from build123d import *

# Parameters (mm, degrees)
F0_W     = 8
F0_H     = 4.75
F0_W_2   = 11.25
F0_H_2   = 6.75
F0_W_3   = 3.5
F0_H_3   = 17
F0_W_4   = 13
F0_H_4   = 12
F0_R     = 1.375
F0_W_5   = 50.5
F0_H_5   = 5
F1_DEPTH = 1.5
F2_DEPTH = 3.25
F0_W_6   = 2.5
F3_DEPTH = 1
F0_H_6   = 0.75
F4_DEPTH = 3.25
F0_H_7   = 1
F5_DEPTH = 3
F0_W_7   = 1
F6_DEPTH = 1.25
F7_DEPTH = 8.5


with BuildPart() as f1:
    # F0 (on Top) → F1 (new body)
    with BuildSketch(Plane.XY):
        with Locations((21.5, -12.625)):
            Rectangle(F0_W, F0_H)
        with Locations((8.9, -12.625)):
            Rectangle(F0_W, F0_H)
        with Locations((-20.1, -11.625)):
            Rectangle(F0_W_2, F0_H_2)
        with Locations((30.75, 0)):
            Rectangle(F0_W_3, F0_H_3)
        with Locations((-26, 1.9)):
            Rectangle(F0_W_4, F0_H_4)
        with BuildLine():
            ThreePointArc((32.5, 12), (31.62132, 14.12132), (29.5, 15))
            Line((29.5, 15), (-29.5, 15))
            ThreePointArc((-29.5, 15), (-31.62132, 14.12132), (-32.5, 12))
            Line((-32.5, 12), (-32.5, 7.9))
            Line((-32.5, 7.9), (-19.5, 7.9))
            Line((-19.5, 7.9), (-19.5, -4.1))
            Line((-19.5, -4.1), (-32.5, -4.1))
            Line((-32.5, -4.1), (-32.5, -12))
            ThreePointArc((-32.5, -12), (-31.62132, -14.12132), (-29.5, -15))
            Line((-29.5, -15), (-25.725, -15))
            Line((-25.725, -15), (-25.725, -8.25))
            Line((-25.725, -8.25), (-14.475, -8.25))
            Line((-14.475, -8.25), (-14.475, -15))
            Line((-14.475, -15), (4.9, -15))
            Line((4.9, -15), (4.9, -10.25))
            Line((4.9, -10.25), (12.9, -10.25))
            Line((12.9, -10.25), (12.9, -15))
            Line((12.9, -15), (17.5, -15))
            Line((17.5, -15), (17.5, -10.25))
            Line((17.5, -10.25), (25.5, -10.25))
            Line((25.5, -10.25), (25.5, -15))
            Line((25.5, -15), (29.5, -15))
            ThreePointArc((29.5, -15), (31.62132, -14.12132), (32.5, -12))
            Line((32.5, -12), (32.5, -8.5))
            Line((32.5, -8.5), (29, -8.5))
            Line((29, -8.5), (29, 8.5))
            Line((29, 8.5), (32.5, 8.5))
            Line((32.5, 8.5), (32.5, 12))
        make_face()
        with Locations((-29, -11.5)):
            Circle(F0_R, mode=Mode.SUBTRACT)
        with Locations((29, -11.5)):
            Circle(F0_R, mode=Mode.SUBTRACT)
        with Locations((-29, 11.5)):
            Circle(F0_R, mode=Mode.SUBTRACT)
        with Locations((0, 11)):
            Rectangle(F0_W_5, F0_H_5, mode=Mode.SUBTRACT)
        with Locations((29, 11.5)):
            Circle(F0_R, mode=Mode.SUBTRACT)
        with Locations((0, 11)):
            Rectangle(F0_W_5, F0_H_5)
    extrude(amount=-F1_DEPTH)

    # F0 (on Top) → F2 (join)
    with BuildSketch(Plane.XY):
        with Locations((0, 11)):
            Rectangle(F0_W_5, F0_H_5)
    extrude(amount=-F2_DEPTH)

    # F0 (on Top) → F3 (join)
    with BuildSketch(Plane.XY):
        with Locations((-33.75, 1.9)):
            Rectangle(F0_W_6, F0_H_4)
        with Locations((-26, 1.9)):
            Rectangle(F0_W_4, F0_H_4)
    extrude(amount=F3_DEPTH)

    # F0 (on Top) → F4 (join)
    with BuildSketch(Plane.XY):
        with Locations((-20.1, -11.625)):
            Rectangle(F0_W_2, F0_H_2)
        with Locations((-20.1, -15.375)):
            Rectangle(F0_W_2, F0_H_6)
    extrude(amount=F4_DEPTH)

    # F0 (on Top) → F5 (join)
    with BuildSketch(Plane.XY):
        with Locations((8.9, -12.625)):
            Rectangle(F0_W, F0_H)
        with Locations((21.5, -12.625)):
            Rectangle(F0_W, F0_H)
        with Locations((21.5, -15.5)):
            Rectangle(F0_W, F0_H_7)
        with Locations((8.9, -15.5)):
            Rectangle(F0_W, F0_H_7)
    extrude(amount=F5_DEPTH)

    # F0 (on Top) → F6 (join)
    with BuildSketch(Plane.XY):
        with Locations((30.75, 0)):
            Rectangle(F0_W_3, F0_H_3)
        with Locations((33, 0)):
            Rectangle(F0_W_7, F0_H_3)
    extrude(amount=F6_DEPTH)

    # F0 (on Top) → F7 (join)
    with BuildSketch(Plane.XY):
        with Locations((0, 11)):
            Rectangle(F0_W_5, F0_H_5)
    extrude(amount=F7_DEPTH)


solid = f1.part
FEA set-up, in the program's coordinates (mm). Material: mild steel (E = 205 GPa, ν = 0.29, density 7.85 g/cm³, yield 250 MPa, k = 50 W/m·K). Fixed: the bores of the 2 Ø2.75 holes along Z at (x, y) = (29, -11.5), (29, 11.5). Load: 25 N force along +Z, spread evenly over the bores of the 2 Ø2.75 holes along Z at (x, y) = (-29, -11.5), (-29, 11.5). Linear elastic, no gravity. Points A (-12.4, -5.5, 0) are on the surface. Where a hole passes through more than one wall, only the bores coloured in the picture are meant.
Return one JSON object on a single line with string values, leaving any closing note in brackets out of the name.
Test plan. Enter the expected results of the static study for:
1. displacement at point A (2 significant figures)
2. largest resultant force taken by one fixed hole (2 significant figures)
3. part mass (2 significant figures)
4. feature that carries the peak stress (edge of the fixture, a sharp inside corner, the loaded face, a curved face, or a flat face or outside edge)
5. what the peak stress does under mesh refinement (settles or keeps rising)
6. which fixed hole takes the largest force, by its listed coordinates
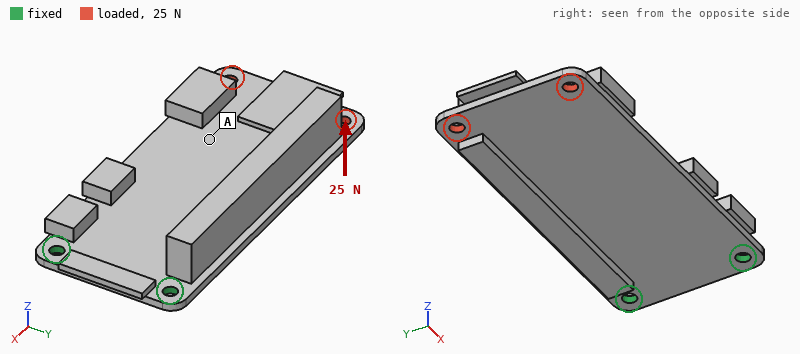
{"displacement at point A": "0.20 mm", "largest resultant force taken by one fixed hole": "21 N", "part mass": "49 g", "feature that carries the peak stress": "edge of the fixture", "what the peak stress does under mesh refinement": "keeps rising", "which fixed hole takes the largest force, by its listed coordinates": "(29, -11.5)"}
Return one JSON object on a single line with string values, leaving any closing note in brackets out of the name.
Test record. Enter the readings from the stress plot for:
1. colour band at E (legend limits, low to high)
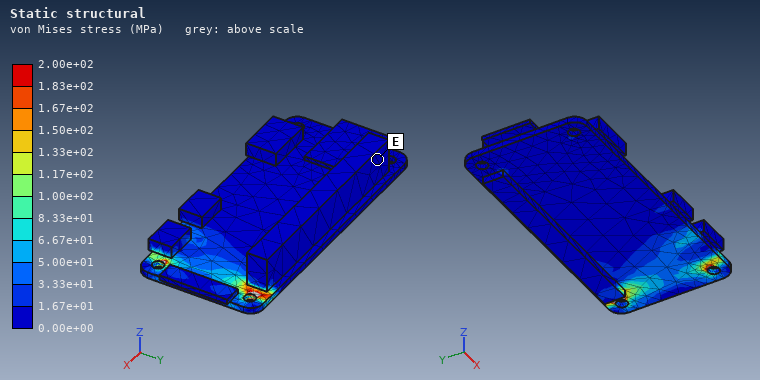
{"colour band at E": "0.00e+00 to 1.67e+01 MPa"}
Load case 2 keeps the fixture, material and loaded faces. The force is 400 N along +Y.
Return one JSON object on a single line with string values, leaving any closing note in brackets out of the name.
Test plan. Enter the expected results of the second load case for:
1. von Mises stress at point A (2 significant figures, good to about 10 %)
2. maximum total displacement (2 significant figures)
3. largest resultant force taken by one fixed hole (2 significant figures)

{"von Mises stress at point A": "20 MPa", "maximum total displacement": "39 µm", "largest resultant force taken by one fixed hole": "1.0 kN"}
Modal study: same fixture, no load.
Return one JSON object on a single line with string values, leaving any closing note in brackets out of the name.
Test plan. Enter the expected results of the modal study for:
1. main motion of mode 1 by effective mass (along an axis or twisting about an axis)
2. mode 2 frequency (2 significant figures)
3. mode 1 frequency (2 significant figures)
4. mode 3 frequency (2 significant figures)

{"main motion of mode 1 by effective mass": "along Z", "mode 2 frequency": "1700 Hz", "mode 1 frequency": "360 Hz", "mode 3 frequency": "3900 Hz"}
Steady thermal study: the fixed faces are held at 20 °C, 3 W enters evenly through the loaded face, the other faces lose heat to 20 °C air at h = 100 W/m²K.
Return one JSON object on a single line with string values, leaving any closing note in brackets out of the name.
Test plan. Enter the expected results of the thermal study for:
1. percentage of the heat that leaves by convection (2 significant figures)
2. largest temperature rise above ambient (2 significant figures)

{"percentage of the heat that leaves by convection": "91 %", "largest temperature rise above ambient": "22 K"}
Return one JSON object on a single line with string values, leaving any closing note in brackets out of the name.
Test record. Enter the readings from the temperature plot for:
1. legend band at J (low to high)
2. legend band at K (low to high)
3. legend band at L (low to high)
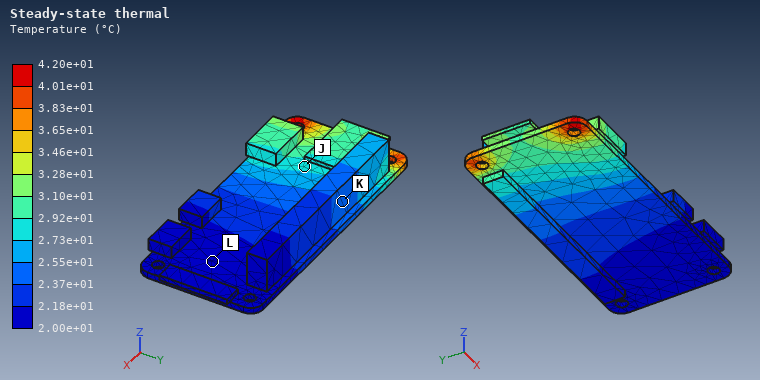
{"legend band at J": "2.73e+01 to 2.92e+01 °C", "legend band at K": "2.37e+01 to 2.55e+01 °C", "legend band at L": "2.00e+01 to 2.18e+01 °C"}
